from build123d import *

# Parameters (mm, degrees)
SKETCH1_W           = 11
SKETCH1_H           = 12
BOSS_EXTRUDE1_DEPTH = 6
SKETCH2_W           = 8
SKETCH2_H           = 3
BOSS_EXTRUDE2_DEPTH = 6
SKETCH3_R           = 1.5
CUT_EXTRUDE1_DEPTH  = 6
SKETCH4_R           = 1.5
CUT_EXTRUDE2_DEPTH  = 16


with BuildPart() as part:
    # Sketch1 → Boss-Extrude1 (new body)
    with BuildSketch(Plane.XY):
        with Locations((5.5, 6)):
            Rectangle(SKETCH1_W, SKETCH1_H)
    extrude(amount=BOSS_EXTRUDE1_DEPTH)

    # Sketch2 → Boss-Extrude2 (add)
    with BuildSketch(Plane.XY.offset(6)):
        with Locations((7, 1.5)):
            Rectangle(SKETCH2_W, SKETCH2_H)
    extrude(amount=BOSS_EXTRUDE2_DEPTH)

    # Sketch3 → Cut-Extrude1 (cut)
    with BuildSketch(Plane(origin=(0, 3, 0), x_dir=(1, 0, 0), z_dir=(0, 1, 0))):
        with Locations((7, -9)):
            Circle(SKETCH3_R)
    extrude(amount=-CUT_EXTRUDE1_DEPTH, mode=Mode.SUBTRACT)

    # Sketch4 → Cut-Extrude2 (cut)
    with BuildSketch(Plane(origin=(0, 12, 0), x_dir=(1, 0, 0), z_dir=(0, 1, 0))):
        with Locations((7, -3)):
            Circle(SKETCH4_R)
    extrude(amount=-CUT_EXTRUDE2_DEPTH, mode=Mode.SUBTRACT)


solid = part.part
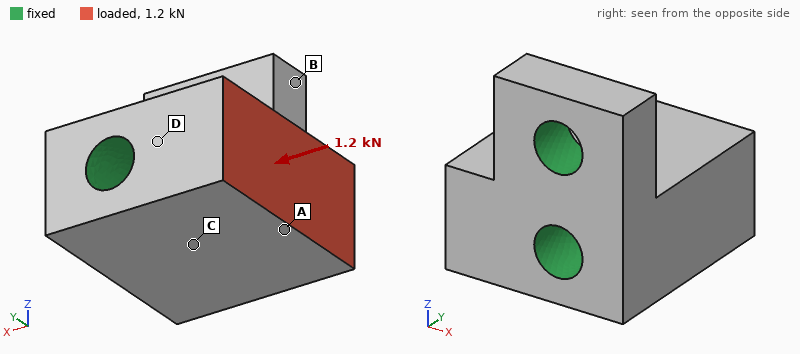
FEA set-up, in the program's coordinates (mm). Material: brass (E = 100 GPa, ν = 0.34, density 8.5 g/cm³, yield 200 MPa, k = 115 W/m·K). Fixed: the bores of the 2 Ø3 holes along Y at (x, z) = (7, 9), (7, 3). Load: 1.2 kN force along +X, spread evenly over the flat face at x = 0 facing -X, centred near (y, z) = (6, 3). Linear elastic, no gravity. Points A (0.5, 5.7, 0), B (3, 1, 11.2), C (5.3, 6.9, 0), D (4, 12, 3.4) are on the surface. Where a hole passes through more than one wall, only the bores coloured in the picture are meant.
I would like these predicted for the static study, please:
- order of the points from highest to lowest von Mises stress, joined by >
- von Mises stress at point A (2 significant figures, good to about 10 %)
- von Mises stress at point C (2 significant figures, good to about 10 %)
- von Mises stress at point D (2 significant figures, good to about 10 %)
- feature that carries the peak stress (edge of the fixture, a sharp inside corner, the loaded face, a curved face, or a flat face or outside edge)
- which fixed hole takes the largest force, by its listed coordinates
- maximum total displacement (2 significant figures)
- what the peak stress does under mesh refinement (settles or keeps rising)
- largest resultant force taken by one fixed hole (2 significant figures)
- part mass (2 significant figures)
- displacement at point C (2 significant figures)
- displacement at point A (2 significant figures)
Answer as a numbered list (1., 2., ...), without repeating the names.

1. D > A > C > B
2. 17 MPa
3. 8.9 MPa
4. 21 MPa
5. edge of the fixture
6. (7, 3)
7. 1.3 µm
8. keeps rising
9. 1.2 kN
10. 7.1 g
11. 0.39 µm
12. 1.0 µm
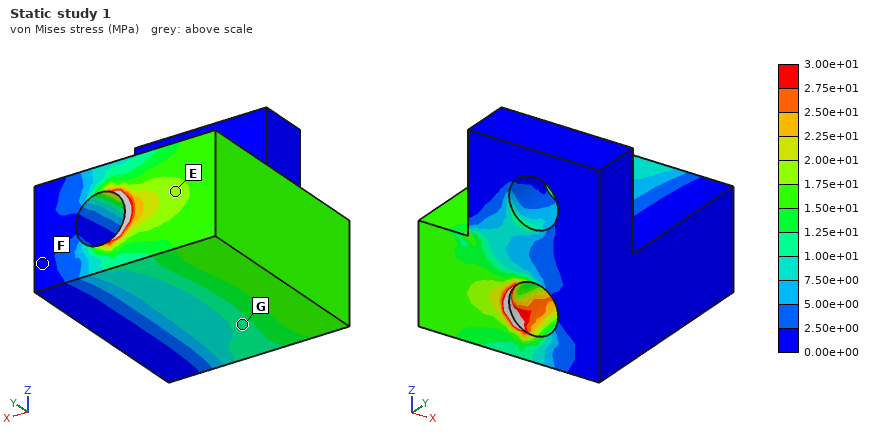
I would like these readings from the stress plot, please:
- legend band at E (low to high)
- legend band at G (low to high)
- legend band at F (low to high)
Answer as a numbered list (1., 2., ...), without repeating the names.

1. 1.75e+01 to 2.00e+01 MPa
2. 1.00e+01 to 1.25e+01 MPa
3. 0.00e+00 to 2.50e+00 MPa
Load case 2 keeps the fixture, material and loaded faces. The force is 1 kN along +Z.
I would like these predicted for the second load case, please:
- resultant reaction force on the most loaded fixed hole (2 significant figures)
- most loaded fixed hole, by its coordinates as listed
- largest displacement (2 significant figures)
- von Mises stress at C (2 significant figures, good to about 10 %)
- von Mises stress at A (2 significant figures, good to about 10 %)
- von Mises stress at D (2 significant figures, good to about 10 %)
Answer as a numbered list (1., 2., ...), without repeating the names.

1. 810 N
2. (7, 3)
3. 8.8 µm
4. 53 MPa
5. 18 MPa
6. 38 MPa
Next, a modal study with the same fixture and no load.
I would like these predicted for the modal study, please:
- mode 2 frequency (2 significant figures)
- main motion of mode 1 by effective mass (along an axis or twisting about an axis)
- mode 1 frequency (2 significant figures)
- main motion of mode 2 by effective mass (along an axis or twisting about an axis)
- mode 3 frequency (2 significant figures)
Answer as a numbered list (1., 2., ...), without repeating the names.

1. 72 kHz
2. along Z
3. 52 kHz
4. along Y
5. 76 kHz
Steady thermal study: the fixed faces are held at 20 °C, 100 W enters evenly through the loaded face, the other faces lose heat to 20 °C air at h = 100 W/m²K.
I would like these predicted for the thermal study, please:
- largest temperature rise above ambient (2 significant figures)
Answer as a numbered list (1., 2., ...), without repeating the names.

1. 72 K
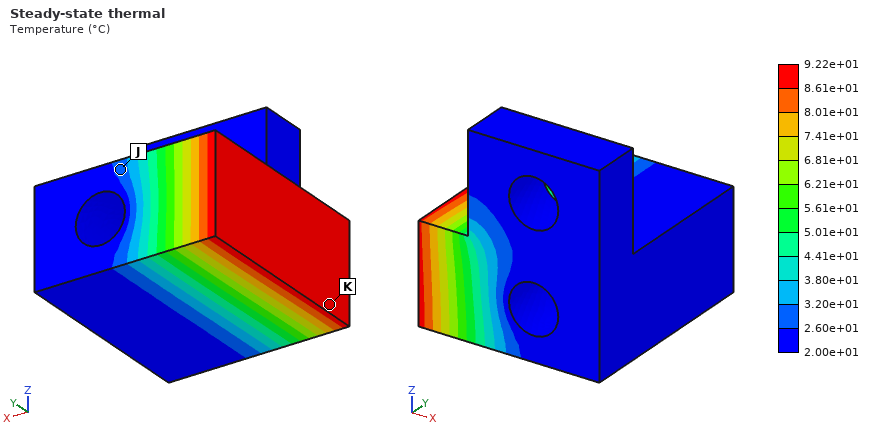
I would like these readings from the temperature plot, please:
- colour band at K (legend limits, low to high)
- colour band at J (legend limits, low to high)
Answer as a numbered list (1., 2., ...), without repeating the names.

1. 8.61e+01 to 9.22e+01 °C
2. 2.60e+01 to 3.20e+01 °C
